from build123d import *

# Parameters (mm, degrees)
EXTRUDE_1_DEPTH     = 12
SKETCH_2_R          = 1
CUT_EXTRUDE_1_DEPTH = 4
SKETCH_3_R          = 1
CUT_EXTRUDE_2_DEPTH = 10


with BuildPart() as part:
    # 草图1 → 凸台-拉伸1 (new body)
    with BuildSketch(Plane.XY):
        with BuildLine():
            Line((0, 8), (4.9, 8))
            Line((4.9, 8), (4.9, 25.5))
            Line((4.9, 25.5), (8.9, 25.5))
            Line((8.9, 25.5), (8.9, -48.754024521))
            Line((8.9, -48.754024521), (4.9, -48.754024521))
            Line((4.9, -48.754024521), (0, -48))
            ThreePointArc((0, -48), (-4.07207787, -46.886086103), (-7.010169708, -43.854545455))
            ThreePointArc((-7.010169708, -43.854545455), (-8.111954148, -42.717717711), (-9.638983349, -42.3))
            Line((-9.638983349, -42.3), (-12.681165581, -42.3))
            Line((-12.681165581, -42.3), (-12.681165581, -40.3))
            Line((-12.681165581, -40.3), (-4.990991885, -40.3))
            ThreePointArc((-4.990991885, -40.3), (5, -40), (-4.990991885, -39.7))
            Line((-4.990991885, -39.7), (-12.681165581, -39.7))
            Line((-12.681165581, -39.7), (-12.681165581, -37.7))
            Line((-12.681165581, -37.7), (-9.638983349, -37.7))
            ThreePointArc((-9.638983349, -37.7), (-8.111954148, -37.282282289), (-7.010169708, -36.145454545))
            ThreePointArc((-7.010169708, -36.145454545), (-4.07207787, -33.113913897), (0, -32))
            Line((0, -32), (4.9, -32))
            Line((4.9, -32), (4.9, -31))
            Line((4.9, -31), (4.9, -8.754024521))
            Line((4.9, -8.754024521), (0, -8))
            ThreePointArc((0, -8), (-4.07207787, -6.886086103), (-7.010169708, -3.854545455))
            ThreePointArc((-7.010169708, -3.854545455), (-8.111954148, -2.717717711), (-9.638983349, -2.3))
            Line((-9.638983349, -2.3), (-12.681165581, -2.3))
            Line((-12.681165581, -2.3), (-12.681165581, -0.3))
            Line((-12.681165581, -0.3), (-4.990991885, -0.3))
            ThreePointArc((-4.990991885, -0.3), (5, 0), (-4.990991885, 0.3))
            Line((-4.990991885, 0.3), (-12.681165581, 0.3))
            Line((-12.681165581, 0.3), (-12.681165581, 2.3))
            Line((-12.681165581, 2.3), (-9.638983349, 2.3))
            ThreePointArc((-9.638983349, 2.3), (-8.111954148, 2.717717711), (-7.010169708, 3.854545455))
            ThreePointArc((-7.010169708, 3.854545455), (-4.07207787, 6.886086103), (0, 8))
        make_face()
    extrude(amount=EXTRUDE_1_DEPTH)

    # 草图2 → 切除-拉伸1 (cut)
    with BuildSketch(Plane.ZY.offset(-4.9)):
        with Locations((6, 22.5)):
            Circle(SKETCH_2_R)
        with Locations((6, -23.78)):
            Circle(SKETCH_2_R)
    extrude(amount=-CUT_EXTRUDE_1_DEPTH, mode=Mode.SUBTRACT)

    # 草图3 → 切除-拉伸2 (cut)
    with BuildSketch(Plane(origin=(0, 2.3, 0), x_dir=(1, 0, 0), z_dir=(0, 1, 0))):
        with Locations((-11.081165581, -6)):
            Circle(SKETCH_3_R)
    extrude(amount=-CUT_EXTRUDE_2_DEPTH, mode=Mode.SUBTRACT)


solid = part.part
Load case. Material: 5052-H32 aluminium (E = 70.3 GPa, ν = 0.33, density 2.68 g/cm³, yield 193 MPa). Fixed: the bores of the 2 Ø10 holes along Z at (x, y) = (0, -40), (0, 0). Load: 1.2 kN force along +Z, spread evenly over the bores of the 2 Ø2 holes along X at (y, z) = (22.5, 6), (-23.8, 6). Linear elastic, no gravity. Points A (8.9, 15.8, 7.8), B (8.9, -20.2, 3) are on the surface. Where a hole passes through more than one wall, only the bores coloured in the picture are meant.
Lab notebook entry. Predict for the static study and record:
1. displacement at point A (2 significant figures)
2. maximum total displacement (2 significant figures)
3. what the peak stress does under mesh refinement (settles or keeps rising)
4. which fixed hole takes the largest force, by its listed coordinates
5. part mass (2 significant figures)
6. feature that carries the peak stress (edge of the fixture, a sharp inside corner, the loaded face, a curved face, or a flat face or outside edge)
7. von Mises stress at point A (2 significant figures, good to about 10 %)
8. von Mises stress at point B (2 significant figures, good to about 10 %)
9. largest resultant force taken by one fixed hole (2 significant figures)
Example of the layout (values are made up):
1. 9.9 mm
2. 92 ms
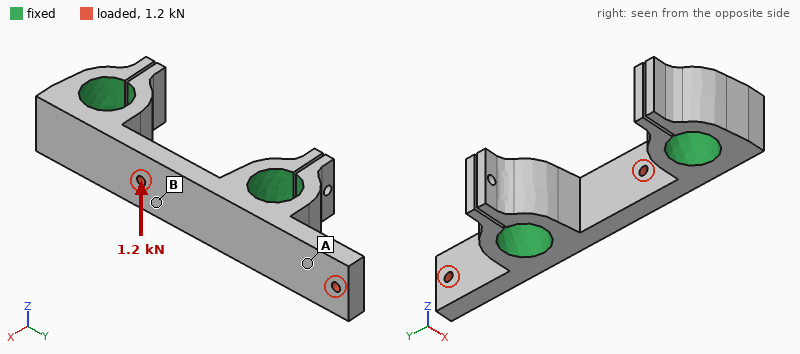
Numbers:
1. 23 µm
2. 58 µm
3. keeps rising
4. (0, 0)
5. 17 g
6. a sharp inside corner
7. 31 MPa
8. 12 MPa
9. 820 N
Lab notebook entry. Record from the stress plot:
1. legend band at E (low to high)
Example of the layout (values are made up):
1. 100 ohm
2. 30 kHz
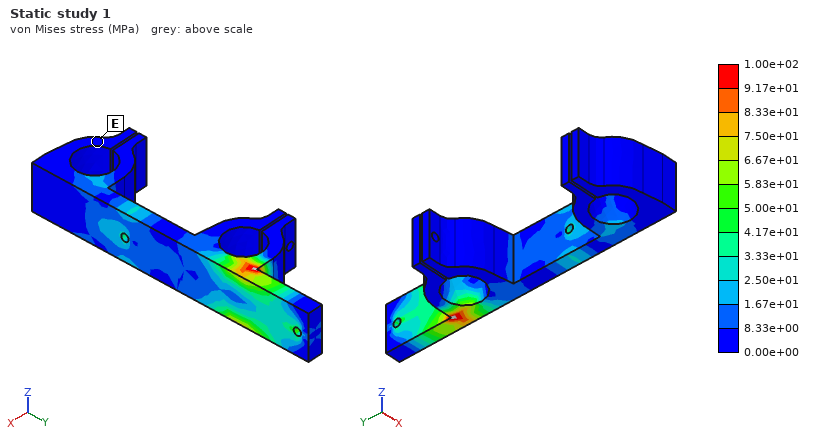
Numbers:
1. 0.00e+00 to 8.33e+00 MPa
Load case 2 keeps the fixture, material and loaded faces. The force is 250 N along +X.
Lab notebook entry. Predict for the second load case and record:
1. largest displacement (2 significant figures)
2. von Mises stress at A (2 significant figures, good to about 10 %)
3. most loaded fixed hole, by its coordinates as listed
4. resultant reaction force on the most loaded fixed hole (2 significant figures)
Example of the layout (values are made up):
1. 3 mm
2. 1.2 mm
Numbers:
1. 56 µm
2. 26 MPa
3. (0, 0)
4. 170 N
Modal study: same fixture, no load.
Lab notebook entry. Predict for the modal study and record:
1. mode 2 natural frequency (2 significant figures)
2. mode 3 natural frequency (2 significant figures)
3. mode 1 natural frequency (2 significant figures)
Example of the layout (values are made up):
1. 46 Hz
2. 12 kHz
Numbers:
1. 17 kHz
2. 25 kHz
3. 8600 Hz
